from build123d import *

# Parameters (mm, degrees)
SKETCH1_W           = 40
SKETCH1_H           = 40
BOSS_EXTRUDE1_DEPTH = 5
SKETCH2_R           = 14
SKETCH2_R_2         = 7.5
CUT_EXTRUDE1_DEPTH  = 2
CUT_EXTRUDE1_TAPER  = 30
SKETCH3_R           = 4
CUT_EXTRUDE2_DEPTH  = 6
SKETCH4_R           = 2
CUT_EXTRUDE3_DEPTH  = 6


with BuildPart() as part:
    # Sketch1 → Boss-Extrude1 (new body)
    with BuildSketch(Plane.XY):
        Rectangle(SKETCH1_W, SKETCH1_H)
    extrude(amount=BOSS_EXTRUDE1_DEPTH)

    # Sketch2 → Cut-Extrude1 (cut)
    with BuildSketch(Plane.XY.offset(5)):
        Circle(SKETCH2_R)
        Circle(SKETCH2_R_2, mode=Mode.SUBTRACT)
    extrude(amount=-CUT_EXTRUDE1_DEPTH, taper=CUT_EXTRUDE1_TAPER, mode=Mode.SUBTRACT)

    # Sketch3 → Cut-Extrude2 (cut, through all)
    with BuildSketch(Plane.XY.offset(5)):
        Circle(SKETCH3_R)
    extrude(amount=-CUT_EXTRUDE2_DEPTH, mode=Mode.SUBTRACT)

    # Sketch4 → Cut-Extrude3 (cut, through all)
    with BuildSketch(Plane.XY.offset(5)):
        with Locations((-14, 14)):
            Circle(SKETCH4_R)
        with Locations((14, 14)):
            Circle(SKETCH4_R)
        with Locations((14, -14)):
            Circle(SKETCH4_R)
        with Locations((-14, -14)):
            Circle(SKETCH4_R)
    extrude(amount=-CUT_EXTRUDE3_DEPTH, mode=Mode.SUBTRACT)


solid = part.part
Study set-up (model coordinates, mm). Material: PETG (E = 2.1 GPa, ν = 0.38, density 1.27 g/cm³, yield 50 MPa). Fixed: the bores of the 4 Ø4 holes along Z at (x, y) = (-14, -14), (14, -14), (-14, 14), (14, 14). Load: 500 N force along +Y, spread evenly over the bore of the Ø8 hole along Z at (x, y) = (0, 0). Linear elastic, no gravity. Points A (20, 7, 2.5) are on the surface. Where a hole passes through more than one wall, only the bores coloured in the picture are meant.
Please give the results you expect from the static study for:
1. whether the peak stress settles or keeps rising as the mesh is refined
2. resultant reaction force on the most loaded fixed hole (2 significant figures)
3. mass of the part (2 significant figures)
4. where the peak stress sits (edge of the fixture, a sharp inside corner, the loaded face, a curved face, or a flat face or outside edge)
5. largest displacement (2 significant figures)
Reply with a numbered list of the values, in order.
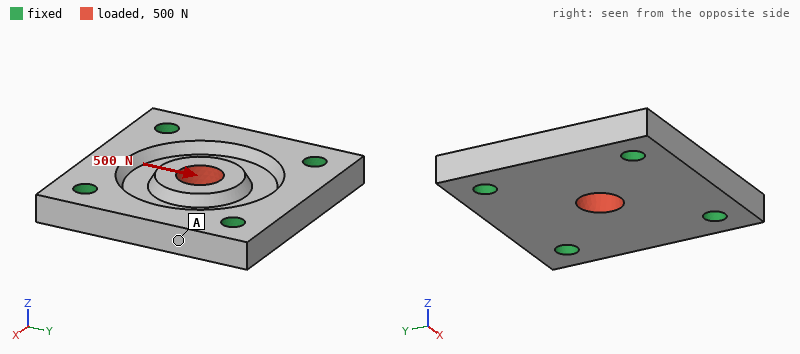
1. keeps rising
2. 140 N
3. 8.6 g
4. edge of the fixture
5. 49 µm
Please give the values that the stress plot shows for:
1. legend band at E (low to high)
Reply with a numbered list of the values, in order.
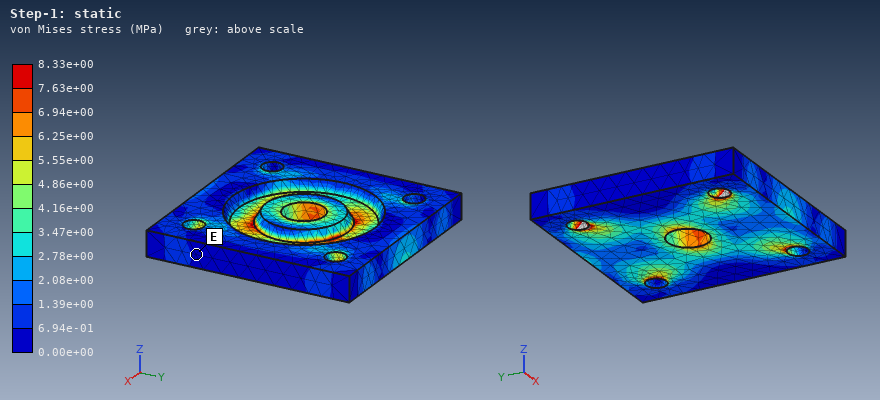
1. 0.00e+00 to 6.94e-01 MPa
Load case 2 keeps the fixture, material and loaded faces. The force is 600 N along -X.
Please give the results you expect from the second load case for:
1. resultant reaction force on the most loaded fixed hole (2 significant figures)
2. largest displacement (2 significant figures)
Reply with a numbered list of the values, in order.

1. 160 N
2. 58 µm
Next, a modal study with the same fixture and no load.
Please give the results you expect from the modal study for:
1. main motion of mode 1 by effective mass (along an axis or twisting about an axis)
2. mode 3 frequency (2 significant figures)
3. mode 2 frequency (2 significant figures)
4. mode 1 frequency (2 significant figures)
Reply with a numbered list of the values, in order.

1. along Z
2. 7900 Hz
3. 7900 Hz
4. 5800 Hz
